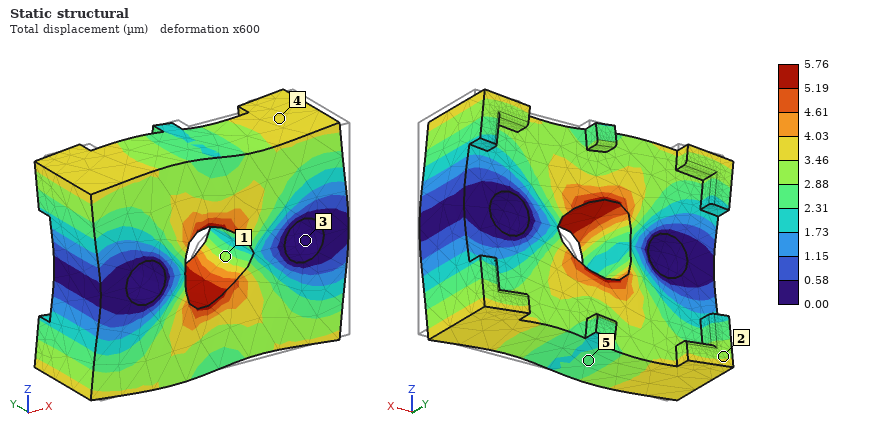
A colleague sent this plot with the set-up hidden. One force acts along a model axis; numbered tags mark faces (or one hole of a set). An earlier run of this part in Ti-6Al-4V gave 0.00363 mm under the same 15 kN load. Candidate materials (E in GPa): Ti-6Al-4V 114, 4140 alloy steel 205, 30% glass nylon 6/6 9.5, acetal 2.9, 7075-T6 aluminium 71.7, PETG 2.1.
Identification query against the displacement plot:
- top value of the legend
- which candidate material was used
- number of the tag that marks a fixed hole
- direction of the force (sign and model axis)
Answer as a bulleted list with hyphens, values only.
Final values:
- 5.76 µm
- 7075-T6 aluminium
- 3
- -X
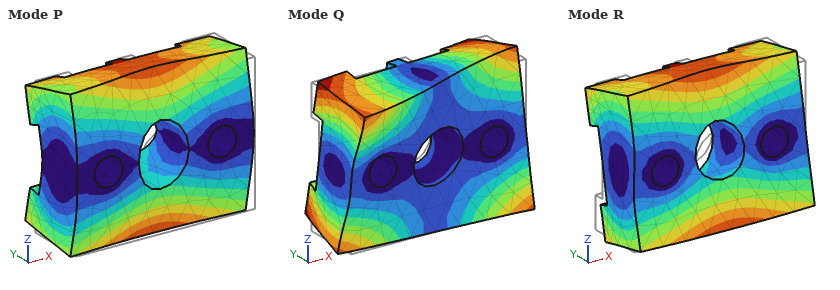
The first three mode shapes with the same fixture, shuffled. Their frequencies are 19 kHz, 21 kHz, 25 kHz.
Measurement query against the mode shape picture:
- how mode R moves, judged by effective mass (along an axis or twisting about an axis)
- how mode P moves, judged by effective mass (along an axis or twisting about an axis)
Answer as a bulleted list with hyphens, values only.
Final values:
- twisting about X
- along Y
